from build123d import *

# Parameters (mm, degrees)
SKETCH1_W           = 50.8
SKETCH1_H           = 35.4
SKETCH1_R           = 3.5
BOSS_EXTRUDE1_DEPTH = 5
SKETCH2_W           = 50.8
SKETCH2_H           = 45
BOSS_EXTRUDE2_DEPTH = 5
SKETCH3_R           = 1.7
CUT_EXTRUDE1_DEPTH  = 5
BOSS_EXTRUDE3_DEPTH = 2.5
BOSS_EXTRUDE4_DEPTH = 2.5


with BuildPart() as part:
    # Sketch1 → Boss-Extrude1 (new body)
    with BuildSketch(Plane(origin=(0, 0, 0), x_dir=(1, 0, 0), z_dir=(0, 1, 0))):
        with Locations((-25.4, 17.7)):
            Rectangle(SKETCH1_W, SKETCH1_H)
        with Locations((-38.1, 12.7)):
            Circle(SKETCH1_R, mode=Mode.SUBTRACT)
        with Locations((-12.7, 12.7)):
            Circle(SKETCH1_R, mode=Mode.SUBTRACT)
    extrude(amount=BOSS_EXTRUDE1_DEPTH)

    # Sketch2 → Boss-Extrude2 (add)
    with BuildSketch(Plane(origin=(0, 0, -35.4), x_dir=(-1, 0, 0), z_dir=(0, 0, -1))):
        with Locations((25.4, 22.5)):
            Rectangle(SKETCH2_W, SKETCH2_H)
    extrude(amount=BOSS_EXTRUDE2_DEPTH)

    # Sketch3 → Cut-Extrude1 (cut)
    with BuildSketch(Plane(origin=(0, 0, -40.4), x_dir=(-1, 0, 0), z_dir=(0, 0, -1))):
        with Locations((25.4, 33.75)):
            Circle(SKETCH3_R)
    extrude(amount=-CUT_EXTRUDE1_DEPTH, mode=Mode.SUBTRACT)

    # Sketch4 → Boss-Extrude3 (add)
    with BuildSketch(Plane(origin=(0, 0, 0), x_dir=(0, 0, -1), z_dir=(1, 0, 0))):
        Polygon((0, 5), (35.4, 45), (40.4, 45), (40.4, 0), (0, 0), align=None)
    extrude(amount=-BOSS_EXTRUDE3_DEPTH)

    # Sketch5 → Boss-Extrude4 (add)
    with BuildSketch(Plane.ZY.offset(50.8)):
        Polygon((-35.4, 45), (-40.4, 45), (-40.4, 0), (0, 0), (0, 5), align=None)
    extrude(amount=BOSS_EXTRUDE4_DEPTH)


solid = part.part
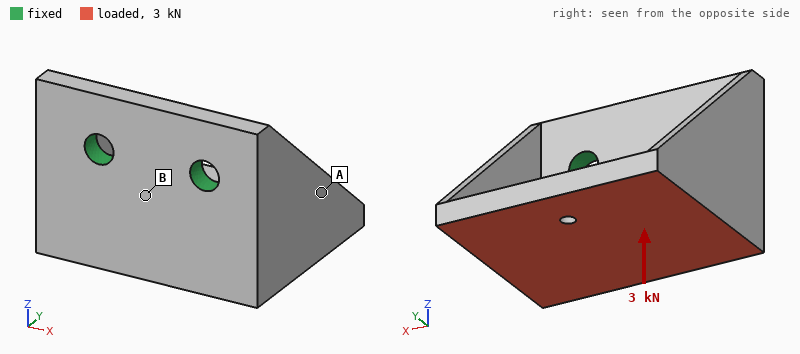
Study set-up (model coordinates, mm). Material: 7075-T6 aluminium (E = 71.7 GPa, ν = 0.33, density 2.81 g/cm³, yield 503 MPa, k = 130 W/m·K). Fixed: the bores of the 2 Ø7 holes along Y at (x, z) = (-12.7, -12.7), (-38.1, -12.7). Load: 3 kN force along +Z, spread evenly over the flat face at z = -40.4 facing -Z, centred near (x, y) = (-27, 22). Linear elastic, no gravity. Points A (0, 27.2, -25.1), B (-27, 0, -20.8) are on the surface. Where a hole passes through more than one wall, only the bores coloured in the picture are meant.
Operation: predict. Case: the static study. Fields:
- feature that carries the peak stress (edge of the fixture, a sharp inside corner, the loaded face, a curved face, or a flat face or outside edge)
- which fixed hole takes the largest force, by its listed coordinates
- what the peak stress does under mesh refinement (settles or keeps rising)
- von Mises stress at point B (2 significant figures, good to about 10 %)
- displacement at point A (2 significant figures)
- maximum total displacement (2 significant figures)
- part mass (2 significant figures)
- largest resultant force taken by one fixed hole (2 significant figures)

edge of the fixture
(-38.1, -12.7)
keeps rising
87 MPa
0.21 mm
0.53 mm
69 g
1.6 kN
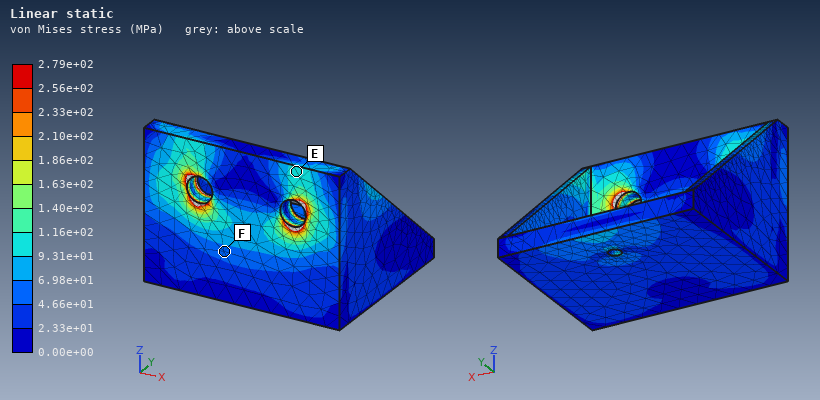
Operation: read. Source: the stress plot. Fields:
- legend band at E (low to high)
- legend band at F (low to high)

9.31e+01 to 1.16e+02 MPa
4.66e+01 to 6.98e+01 MPa
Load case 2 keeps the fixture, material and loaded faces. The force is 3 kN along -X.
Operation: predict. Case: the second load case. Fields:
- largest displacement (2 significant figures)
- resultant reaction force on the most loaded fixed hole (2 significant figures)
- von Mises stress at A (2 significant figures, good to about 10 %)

0.37 mm
3.4 kN
30 MPa
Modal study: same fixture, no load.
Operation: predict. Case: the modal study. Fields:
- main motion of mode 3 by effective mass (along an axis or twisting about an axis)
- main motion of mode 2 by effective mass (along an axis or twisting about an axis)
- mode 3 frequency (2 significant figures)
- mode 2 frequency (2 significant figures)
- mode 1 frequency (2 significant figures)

along Y
along X
6100 Hz
2400 Hz
2000 Hz
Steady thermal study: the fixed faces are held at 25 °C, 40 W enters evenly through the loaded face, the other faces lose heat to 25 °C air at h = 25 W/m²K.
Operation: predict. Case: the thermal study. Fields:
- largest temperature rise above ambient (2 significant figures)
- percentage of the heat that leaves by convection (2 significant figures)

35 K
11 %
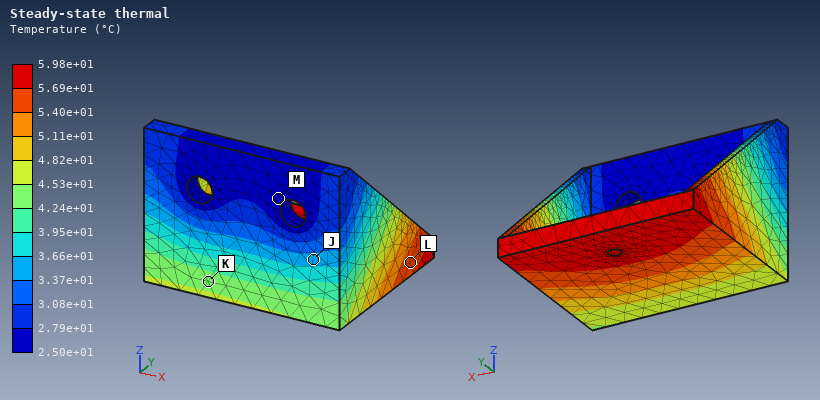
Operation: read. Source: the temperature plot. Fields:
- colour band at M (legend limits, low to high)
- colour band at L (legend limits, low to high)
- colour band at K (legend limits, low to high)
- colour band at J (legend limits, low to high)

2.50e+01 to 2.79e+01 °C
5.40e+01 to 5.69e+01 °C
4.24e+01 to 4.53e+01 °C
3.37e+01 to 3.66e+01 °C
